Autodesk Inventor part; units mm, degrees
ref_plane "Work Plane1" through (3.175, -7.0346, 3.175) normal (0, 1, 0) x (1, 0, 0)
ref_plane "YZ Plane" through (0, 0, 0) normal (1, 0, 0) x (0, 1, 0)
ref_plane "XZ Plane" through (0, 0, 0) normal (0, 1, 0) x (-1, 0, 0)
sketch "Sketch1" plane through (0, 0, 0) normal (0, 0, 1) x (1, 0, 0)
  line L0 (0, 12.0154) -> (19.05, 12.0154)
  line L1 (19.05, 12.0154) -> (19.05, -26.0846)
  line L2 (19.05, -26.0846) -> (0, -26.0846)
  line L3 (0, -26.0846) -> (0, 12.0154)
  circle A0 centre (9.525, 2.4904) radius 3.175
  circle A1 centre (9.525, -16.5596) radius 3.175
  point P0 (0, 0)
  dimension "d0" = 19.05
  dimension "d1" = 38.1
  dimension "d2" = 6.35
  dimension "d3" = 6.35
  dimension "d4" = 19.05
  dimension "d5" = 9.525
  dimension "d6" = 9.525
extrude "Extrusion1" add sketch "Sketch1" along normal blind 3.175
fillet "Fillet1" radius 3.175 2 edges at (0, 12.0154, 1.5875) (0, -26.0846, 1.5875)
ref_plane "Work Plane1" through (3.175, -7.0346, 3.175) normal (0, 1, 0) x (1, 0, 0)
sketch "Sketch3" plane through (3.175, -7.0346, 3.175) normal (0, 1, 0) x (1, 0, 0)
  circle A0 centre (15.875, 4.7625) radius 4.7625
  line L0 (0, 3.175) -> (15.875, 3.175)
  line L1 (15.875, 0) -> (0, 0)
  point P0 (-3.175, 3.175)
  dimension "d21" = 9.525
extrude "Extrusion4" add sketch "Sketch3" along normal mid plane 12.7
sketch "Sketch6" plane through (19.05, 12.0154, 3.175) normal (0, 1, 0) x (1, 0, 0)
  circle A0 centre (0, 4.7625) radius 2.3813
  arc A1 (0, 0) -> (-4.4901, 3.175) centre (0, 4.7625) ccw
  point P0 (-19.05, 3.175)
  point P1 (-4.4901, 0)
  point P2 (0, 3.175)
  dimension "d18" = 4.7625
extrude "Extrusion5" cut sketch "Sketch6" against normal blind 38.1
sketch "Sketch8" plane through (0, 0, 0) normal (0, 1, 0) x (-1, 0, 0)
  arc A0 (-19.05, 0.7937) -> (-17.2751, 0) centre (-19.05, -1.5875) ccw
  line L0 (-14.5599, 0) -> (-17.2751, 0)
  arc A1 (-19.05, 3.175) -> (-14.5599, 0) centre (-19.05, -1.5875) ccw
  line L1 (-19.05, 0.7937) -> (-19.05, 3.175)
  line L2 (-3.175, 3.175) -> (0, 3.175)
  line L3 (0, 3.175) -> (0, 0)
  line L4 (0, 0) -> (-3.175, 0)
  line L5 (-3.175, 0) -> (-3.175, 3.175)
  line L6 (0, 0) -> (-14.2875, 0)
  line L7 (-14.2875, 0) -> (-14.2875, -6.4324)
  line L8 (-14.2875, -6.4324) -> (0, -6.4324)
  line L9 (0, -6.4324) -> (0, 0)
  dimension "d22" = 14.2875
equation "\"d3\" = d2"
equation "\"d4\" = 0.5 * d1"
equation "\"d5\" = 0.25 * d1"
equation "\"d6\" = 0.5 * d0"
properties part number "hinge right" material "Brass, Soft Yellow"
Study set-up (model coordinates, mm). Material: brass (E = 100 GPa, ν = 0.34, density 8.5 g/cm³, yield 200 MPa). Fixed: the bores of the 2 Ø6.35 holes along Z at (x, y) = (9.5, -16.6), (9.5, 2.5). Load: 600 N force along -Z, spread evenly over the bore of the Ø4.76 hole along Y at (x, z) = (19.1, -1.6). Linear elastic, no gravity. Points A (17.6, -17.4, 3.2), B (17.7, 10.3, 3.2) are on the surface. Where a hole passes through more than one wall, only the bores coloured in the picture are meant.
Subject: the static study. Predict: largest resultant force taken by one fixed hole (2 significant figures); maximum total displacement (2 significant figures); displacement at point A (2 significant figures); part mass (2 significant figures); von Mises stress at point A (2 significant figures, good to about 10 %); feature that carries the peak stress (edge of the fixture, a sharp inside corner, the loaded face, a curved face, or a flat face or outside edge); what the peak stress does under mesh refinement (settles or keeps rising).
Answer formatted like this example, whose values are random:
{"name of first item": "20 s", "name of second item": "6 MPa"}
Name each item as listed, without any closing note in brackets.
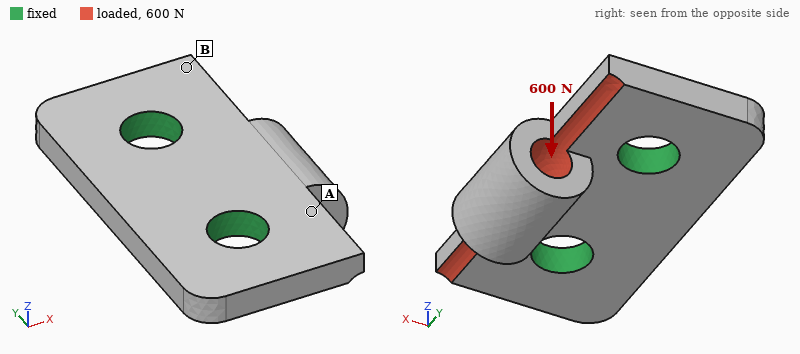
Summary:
{"largest resultant force taken by one fixed hole": "300 N", "maximum total displacement": "31 µm", "displacement at point A": "6.4 µm", "part mass": "22 g", "von Mises stress at point A": "33 MPa", "feature that carries the peak stress": "edge of the fixture", "what the peak stress does under mesh refinement": "keeps rising"}
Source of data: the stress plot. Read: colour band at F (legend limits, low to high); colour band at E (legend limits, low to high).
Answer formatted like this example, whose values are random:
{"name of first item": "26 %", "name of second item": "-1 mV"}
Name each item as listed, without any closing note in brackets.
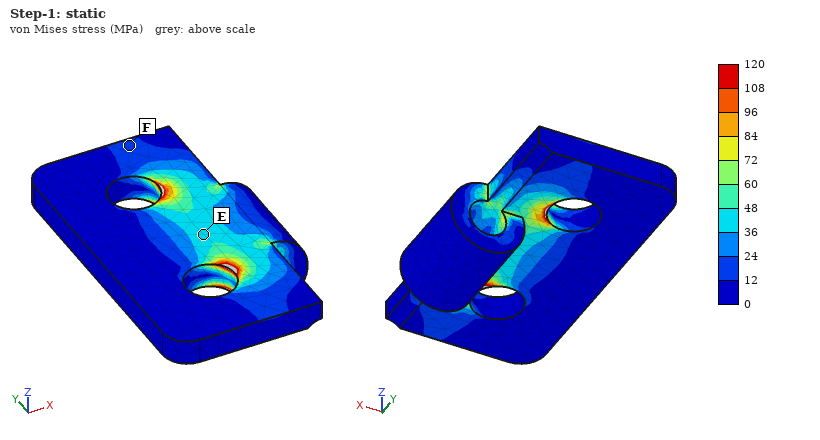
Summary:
{"colour band at F": "12 to 24 MPa", "colour band at E": "36 to 48 MPa"}
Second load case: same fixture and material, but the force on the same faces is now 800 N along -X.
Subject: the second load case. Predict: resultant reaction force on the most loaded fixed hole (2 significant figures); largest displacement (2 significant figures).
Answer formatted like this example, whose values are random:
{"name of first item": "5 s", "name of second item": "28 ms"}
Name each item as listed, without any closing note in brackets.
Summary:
{"resultant reaction force on the most loaded fixed hole": "410 N", "largest displacement": "24 µm"}
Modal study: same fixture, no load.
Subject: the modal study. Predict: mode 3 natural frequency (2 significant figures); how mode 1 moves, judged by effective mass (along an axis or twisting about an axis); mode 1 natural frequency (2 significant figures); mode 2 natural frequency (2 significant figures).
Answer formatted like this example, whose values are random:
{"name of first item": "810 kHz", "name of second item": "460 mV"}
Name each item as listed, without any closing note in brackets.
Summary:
{"mode 3 natural frequency": "23 kHz", "how mode 1 moves, judged by effective mass": "along Z", "mode 1 natural frequency": "8800 Hz", "mode 2 natural frequency": "22 kHz"}
